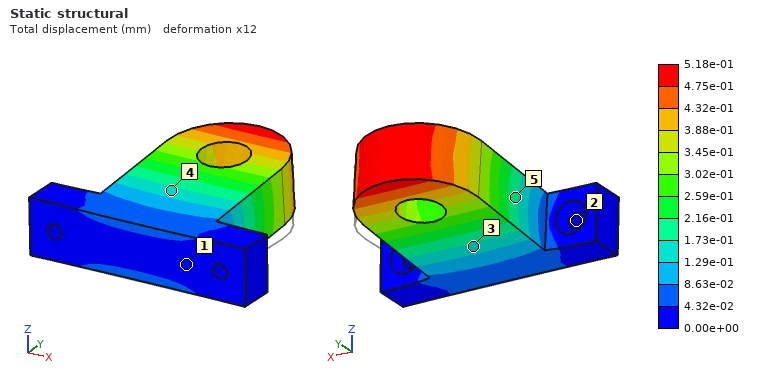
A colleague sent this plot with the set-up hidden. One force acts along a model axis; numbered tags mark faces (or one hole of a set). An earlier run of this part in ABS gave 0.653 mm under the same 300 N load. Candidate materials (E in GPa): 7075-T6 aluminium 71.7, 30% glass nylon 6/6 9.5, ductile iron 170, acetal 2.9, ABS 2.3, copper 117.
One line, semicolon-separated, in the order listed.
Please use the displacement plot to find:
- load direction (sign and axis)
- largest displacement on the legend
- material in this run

+Z; 5.18e-01 mm; acetal
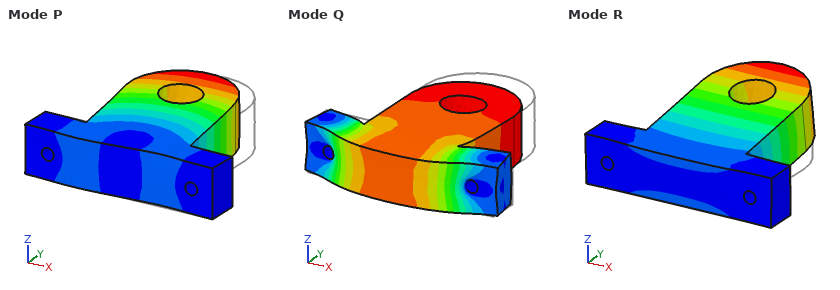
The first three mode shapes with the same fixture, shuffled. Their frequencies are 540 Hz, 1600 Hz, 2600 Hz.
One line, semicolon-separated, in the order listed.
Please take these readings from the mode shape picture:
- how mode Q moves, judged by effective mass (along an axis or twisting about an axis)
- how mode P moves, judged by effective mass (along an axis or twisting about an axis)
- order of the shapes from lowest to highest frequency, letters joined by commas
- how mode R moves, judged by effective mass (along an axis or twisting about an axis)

along Y; along X; R, P, Q; along Z
